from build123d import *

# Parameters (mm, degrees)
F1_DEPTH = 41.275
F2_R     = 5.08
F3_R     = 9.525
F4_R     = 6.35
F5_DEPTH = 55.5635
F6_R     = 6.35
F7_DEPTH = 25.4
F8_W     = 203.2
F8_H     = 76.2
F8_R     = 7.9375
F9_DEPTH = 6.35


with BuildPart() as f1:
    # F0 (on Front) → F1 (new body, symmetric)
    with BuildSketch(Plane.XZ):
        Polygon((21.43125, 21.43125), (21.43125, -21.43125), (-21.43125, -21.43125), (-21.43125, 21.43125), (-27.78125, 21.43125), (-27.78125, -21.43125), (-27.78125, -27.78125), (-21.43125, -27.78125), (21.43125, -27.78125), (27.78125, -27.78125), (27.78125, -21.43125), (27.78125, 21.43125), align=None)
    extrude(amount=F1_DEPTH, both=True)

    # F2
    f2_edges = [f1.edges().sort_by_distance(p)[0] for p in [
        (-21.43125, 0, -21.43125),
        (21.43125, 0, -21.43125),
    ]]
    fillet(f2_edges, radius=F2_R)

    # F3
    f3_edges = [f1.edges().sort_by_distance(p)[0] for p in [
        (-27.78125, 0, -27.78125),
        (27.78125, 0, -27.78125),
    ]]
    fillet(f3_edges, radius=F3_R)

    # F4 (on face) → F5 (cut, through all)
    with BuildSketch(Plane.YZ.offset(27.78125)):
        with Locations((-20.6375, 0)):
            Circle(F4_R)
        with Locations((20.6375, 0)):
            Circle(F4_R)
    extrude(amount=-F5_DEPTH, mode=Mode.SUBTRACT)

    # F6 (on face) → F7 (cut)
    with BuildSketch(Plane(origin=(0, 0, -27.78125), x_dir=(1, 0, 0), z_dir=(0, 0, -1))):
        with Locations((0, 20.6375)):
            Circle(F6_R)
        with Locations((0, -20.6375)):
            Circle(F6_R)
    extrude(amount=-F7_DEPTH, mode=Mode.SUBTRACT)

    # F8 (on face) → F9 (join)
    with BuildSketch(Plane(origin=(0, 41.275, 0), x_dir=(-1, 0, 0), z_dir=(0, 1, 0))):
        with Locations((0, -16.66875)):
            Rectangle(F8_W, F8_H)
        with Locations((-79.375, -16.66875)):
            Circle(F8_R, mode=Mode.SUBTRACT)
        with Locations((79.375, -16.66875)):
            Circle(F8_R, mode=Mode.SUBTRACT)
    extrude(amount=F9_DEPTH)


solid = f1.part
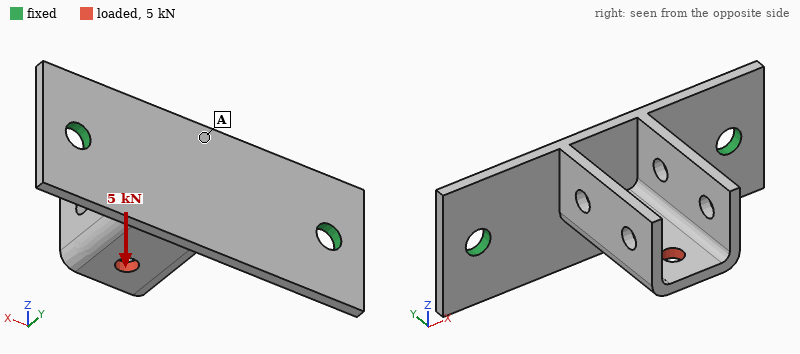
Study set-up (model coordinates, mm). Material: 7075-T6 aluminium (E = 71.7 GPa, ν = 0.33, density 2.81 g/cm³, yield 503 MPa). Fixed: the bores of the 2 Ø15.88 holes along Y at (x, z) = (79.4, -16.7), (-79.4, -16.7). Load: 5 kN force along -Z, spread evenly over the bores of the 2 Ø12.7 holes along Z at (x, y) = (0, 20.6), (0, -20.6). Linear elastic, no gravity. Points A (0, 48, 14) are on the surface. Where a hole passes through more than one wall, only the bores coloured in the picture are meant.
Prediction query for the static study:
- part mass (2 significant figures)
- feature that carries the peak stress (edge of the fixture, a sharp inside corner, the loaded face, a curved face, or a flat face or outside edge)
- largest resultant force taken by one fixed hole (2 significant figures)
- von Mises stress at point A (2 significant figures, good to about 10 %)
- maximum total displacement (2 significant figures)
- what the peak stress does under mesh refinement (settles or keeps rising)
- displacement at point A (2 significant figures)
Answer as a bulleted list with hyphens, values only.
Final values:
- 460 g
- edge of the fixture
- 2.5 kN
- 46 MPa
- 2.6 mm
- keeps rising
- 0.82 mm
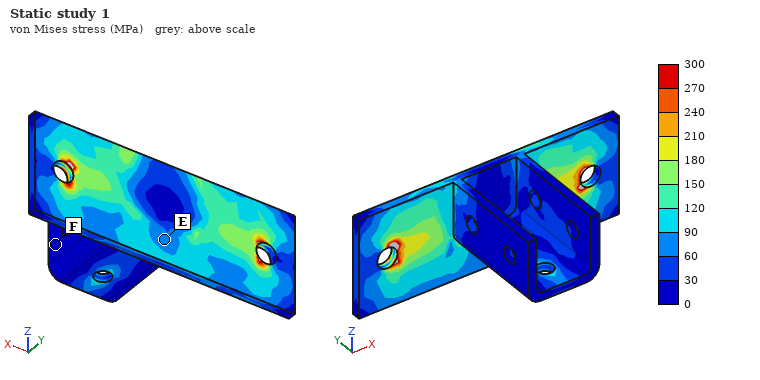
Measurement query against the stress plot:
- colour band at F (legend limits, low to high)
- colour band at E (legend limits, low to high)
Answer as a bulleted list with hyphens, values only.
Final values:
- 0 to 30 MPa
- 60 to 90 MPa
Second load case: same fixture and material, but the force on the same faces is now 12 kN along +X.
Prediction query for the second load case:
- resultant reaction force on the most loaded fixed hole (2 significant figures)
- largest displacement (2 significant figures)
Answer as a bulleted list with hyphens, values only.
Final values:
- 7.7 kN
- 1.4 mm
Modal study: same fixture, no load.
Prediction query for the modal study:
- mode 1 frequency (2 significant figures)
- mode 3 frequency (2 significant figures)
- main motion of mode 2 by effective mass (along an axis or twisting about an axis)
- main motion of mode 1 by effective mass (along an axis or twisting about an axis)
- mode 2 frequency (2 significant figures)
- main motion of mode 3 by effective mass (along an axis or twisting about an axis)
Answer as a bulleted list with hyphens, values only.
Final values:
- 580 Hz
- 1100 Hz
- along Y
- along Z
- 1100 Hz
- along X
